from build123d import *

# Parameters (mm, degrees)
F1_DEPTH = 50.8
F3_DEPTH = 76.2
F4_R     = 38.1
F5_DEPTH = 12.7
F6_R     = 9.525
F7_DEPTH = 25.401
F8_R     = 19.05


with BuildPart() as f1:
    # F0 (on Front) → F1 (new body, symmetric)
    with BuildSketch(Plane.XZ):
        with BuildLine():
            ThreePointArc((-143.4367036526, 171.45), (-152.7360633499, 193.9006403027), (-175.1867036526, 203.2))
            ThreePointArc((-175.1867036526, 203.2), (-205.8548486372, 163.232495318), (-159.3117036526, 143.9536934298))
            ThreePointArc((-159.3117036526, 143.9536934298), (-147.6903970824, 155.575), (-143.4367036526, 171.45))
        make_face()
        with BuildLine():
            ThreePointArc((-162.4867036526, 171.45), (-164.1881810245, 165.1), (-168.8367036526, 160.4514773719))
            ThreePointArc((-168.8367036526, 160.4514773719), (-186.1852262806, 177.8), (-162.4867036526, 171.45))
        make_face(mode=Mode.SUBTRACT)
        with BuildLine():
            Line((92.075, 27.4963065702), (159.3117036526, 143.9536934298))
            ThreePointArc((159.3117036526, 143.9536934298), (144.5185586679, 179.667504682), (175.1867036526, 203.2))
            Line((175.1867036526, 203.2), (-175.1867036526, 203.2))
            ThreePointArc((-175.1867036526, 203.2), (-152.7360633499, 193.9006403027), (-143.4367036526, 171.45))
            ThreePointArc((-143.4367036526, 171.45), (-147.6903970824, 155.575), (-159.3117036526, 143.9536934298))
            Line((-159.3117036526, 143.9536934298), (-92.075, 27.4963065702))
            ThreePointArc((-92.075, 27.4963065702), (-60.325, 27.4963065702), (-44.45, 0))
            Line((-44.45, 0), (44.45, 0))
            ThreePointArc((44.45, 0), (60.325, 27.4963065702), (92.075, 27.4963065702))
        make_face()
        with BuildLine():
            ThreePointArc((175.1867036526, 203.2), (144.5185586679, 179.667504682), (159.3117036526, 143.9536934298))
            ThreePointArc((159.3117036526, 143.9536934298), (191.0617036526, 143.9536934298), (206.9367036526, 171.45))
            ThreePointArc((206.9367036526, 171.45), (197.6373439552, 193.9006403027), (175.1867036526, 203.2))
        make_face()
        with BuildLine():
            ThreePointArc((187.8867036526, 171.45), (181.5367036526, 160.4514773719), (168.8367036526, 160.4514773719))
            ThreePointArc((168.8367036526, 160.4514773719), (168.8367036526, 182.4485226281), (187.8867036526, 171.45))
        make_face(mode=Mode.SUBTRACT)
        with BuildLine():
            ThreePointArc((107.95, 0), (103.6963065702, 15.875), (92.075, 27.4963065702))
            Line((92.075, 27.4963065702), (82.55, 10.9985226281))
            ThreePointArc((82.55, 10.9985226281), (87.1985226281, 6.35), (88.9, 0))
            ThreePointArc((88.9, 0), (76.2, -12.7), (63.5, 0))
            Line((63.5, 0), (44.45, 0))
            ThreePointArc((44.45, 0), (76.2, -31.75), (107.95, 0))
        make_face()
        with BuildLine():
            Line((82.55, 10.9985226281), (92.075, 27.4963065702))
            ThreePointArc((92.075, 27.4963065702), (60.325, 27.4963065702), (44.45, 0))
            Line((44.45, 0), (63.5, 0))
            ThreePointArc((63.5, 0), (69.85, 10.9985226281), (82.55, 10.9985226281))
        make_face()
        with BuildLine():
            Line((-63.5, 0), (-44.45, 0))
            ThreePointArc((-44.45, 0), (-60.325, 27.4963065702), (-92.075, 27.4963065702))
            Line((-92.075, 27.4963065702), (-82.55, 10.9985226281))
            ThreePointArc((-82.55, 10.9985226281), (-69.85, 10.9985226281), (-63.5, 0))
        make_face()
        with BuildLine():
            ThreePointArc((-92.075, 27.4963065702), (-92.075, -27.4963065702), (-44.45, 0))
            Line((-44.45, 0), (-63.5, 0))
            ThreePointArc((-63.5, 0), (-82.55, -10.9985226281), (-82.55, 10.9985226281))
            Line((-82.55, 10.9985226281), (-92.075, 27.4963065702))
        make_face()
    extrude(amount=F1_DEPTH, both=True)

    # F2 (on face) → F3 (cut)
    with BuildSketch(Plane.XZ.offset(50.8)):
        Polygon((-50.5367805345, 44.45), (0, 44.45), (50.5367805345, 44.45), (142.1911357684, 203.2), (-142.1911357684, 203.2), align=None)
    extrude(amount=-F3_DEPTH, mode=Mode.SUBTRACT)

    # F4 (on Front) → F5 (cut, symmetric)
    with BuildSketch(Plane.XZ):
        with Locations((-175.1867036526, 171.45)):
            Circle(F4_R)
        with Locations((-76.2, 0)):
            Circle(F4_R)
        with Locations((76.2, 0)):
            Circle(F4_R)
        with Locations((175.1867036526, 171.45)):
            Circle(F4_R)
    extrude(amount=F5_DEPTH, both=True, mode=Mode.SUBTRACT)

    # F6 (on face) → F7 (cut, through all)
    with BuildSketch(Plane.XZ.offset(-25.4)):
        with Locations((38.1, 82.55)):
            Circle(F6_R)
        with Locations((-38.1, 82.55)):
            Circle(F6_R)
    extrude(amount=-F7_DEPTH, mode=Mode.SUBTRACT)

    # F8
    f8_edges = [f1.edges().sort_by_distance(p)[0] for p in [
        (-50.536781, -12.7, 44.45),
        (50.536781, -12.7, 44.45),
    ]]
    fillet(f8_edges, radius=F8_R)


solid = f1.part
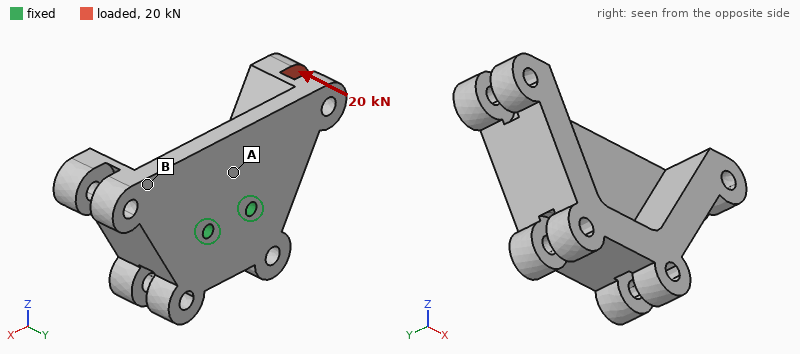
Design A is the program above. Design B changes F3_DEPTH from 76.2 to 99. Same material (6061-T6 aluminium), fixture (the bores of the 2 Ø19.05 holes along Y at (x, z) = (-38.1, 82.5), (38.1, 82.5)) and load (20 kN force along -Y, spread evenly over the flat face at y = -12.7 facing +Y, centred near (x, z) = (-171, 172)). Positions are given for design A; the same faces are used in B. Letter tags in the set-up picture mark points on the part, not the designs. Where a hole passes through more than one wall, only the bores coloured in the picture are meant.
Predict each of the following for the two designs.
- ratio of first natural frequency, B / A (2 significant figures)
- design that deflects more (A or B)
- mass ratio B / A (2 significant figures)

0.060
B
0.80
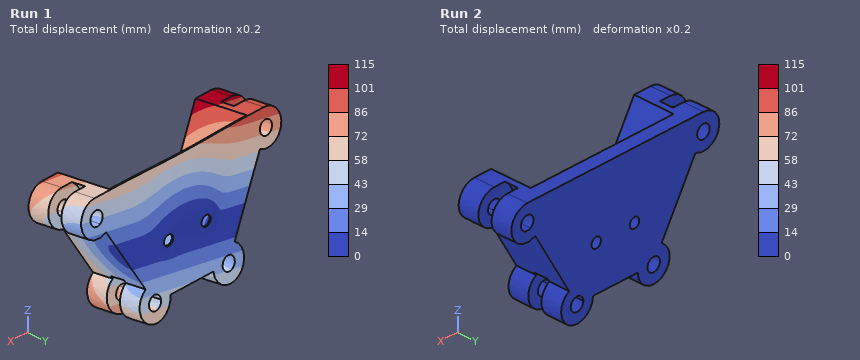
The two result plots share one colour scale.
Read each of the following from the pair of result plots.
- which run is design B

Run 1
